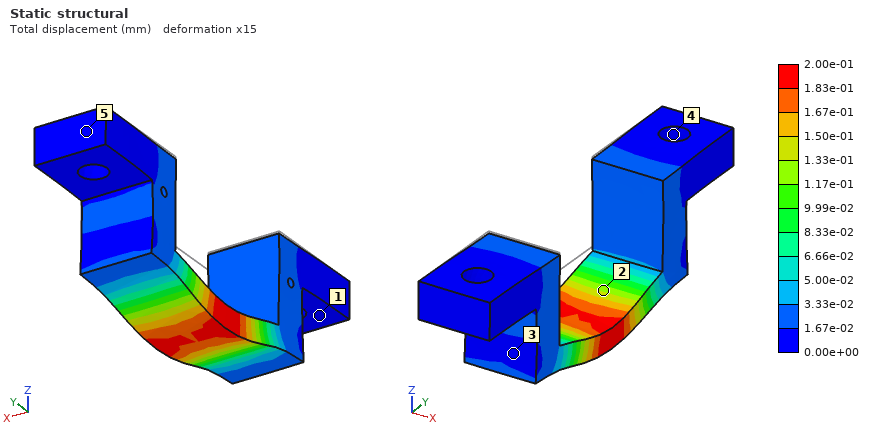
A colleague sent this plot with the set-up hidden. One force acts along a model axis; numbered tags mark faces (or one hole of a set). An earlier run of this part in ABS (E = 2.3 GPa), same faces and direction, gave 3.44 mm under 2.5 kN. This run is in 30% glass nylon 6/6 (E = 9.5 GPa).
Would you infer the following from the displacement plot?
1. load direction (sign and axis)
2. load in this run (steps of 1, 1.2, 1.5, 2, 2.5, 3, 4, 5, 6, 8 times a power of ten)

-Z
600 N
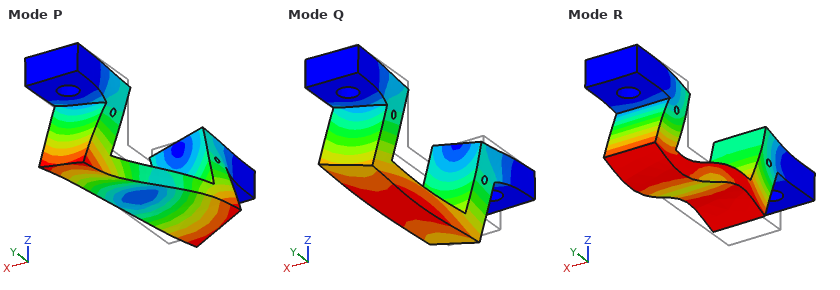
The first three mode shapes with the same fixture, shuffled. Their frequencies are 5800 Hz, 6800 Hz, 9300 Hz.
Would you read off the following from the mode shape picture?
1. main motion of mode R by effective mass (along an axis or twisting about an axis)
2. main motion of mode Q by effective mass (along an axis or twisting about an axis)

along Y
along X
